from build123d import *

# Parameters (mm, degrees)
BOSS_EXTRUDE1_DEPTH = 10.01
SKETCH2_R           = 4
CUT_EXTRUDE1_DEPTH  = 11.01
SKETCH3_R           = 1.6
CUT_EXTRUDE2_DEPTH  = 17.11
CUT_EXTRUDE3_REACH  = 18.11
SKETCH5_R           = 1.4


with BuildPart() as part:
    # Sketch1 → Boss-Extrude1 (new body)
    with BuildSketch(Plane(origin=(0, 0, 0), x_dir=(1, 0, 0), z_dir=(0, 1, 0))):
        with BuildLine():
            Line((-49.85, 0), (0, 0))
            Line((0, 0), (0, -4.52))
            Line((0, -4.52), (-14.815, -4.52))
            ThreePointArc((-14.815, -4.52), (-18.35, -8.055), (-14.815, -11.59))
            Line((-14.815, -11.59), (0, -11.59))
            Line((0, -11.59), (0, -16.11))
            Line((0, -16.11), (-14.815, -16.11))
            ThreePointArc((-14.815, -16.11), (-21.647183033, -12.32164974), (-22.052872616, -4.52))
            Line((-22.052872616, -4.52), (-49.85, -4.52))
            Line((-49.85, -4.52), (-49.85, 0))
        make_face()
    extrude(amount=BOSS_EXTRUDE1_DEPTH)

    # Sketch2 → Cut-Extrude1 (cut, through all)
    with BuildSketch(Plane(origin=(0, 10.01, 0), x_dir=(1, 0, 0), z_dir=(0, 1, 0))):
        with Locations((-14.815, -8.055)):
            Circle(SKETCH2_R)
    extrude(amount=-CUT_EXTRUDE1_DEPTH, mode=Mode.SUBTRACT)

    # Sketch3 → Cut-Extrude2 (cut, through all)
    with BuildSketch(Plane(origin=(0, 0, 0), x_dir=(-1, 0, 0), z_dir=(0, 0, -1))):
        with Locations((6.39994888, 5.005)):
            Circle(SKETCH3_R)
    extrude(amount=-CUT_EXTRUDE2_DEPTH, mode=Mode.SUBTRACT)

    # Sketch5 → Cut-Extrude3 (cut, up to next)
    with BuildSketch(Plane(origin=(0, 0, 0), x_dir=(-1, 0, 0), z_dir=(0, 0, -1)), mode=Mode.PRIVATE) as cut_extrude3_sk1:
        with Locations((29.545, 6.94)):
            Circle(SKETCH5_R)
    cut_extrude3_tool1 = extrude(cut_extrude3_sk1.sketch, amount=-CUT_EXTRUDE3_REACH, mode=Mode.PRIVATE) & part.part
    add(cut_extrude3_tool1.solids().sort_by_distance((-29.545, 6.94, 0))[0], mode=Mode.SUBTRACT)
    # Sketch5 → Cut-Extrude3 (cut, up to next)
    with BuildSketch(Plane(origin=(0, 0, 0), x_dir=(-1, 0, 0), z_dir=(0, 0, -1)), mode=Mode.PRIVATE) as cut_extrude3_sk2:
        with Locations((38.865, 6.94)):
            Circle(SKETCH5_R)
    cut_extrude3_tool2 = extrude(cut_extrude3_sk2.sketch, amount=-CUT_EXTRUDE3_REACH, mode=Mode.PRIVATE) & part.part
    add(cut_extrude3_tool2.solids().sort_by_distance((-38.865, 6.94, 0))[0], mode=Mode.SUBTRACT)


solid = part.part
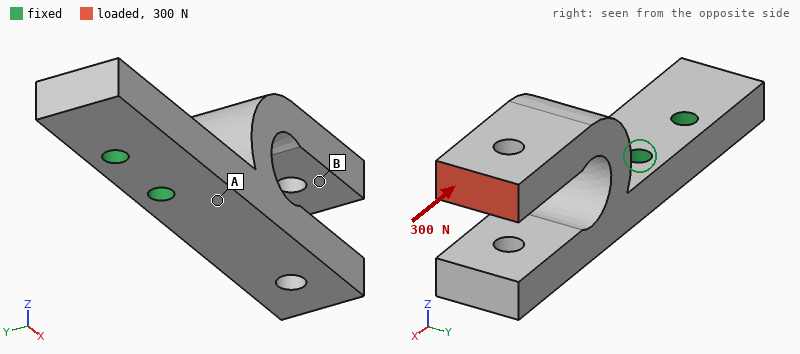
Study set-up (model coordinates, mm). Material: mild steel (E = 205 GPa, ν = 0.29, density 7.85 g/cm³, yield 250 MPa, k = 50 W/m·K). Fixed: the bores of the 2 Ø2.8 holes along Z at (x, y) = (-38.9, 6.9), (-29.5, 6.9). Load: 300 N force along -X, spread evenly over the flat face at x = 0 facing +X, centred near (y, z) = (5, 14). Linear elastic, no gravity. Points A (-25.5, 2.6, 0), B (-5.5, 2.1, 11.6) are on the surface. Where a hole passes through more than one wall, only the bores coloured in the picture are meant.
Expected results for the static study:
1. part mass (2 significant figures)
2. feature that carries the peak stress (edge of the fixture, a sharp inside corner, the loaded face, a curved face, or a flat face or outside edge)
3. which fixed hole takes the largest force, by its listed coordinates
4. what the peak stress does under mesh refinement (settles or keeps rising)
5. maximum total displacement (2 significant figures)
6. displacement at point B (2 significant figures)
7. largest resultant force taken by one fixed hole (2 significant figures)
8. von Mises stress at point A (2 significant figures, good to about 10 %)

26 g
edge of the fixture
(-29.5, 6.9)
keeps rising
90 µm
66 µm
260 N
82 MPa
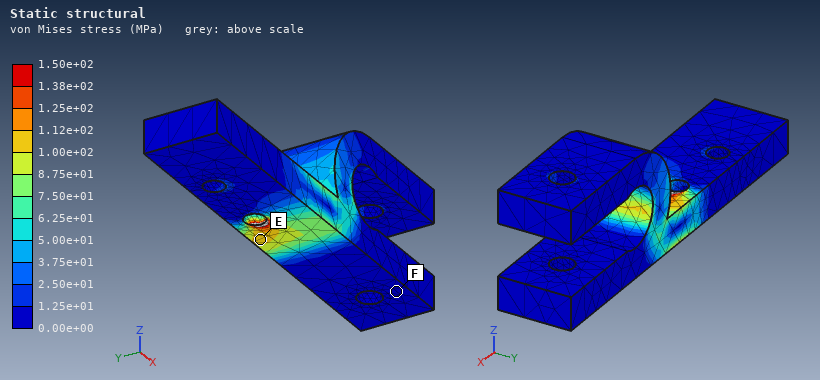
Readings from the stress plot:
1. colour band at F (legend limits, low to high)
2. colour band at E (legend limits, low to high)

0.00e+00 to 1.25e+01 MPa
1.00e+02 to 1.12e+02 MPa
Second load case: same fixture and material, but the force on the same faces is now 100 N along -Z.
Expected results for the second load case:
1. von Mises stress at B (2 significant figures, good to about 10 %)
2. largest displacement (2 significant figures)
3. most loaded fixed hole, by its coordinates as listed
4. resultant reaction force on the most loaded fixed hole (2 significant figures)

22 MPa
99 µm
(-29.5, 6.9)
170 N
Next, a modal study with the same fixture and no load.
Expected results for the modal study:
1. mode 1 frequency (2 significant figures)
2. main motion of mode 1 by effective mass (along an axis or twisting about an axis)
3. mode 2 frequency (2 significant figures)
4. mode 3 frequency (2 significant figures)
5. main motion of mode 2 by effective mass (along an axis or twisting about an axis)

2700 Hz
along Z
4300 Hz
6600 Hz
along Y
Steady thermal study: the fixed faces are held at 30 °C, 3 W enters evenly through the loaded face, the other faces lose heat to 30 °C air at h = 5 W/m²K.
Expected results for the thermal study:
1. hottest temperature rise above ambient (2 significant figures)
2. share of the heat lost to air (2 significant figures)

52 K
5.9 %
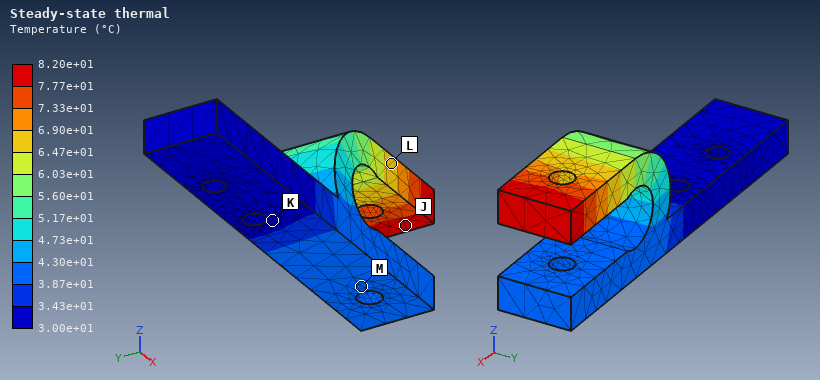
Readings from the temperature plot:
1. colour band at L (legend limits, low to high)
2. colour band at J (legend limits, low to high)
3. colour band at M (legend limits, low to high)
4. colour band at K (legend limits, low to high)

6.47e+01 to 6.90e+01 °C
7.77e+01 to 8.20e+01 °C
3.87e+01 to 4.30e+01 °C
3.00e+01 to 3.43e+01 °C
